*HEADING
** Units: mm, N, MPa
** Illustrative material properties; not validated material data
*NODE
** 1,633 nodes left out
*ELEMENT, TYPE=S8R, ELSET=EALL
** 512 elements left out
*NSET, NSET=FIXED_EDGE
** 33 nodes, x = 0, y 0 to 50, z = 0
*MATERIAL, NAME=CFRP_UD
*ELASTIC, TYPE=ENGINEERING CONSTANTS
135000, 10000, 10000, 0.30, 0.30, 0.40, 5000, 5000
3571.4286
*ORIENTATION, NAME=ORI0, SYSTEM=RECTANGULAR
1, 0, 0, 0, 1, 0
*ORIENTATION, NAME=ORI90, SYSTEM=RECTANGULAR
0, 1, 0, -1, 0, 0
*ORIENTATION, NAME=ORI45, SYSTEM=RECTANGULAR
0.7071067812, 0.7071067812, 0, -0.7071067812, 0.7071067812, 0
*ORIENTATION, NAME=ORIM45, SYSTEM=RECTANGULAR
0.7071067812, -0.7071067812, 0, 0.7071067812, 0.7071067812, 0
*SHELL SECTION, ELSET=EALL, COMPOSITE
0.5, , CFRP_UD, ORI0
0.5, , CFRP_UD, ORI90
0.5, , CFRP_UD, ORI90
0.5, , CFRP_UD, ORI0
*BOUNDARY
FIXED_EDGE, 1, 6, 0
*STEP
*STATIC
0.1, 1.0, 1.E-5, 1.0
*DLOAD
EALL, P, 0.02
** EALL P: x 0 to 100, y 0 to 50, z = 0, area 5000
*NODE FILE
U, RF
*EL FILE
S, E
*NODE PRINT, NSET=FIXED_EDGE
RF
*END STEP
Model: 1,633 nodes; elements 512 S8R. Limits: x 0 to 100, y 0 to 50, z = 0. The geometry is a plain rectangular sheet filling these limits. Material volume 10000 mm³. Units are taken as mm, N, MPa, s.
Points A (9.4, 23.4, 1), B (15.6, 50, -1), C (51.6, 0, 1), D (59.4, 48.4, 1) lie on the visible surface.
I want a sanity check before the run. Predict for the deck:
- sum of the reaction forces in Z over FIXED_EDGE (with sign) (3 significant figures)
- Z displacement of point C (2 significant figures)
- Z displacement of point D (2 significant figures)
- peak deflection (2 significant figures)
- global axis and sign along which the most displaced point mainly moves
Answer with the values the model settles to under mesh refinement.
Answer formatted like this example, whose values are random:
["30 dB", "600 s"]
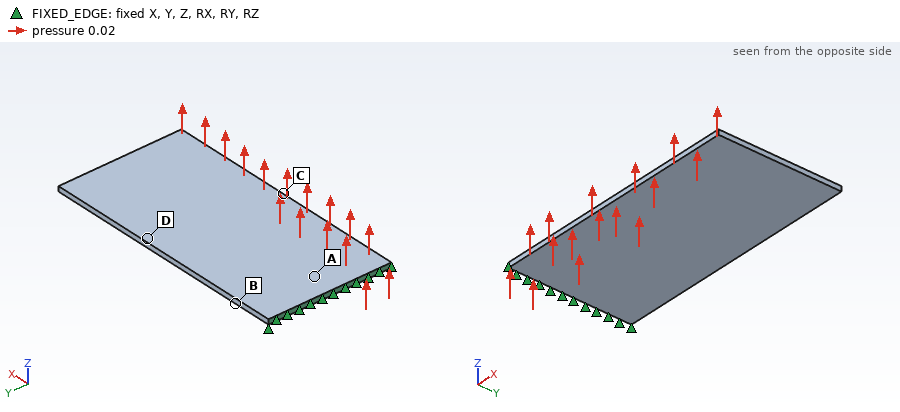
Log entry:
["-100 N", "1.2 mm", "1.5 mm", "3.1 mm", "+Z"]
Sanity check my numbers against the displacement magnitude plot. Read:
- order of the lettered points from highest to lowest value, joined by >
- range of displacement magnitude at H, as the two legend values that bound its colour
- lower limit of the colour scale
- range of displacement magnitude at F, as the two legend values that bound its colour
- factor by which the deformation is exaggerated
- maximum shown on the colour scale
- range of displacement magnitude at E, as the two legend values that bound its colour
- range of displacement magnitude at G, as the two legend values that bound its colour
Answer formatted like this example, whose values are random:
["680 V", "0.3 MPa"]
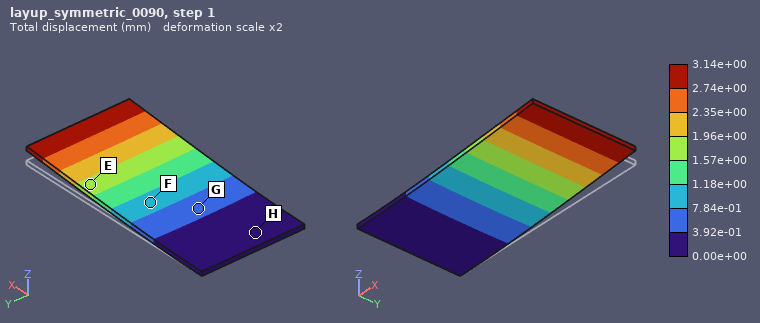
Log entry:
["E > F > G > H", "0.00e+00 to 3.92e-01 mm", "0.00e+00 mm", "7.84e-01 to 1.18e+00 mm", "2", "3.14e+00 mm", "1.57e+00 to 1.96e+00 mm", "3.92e-01 to 7.84e-01 mm"]
